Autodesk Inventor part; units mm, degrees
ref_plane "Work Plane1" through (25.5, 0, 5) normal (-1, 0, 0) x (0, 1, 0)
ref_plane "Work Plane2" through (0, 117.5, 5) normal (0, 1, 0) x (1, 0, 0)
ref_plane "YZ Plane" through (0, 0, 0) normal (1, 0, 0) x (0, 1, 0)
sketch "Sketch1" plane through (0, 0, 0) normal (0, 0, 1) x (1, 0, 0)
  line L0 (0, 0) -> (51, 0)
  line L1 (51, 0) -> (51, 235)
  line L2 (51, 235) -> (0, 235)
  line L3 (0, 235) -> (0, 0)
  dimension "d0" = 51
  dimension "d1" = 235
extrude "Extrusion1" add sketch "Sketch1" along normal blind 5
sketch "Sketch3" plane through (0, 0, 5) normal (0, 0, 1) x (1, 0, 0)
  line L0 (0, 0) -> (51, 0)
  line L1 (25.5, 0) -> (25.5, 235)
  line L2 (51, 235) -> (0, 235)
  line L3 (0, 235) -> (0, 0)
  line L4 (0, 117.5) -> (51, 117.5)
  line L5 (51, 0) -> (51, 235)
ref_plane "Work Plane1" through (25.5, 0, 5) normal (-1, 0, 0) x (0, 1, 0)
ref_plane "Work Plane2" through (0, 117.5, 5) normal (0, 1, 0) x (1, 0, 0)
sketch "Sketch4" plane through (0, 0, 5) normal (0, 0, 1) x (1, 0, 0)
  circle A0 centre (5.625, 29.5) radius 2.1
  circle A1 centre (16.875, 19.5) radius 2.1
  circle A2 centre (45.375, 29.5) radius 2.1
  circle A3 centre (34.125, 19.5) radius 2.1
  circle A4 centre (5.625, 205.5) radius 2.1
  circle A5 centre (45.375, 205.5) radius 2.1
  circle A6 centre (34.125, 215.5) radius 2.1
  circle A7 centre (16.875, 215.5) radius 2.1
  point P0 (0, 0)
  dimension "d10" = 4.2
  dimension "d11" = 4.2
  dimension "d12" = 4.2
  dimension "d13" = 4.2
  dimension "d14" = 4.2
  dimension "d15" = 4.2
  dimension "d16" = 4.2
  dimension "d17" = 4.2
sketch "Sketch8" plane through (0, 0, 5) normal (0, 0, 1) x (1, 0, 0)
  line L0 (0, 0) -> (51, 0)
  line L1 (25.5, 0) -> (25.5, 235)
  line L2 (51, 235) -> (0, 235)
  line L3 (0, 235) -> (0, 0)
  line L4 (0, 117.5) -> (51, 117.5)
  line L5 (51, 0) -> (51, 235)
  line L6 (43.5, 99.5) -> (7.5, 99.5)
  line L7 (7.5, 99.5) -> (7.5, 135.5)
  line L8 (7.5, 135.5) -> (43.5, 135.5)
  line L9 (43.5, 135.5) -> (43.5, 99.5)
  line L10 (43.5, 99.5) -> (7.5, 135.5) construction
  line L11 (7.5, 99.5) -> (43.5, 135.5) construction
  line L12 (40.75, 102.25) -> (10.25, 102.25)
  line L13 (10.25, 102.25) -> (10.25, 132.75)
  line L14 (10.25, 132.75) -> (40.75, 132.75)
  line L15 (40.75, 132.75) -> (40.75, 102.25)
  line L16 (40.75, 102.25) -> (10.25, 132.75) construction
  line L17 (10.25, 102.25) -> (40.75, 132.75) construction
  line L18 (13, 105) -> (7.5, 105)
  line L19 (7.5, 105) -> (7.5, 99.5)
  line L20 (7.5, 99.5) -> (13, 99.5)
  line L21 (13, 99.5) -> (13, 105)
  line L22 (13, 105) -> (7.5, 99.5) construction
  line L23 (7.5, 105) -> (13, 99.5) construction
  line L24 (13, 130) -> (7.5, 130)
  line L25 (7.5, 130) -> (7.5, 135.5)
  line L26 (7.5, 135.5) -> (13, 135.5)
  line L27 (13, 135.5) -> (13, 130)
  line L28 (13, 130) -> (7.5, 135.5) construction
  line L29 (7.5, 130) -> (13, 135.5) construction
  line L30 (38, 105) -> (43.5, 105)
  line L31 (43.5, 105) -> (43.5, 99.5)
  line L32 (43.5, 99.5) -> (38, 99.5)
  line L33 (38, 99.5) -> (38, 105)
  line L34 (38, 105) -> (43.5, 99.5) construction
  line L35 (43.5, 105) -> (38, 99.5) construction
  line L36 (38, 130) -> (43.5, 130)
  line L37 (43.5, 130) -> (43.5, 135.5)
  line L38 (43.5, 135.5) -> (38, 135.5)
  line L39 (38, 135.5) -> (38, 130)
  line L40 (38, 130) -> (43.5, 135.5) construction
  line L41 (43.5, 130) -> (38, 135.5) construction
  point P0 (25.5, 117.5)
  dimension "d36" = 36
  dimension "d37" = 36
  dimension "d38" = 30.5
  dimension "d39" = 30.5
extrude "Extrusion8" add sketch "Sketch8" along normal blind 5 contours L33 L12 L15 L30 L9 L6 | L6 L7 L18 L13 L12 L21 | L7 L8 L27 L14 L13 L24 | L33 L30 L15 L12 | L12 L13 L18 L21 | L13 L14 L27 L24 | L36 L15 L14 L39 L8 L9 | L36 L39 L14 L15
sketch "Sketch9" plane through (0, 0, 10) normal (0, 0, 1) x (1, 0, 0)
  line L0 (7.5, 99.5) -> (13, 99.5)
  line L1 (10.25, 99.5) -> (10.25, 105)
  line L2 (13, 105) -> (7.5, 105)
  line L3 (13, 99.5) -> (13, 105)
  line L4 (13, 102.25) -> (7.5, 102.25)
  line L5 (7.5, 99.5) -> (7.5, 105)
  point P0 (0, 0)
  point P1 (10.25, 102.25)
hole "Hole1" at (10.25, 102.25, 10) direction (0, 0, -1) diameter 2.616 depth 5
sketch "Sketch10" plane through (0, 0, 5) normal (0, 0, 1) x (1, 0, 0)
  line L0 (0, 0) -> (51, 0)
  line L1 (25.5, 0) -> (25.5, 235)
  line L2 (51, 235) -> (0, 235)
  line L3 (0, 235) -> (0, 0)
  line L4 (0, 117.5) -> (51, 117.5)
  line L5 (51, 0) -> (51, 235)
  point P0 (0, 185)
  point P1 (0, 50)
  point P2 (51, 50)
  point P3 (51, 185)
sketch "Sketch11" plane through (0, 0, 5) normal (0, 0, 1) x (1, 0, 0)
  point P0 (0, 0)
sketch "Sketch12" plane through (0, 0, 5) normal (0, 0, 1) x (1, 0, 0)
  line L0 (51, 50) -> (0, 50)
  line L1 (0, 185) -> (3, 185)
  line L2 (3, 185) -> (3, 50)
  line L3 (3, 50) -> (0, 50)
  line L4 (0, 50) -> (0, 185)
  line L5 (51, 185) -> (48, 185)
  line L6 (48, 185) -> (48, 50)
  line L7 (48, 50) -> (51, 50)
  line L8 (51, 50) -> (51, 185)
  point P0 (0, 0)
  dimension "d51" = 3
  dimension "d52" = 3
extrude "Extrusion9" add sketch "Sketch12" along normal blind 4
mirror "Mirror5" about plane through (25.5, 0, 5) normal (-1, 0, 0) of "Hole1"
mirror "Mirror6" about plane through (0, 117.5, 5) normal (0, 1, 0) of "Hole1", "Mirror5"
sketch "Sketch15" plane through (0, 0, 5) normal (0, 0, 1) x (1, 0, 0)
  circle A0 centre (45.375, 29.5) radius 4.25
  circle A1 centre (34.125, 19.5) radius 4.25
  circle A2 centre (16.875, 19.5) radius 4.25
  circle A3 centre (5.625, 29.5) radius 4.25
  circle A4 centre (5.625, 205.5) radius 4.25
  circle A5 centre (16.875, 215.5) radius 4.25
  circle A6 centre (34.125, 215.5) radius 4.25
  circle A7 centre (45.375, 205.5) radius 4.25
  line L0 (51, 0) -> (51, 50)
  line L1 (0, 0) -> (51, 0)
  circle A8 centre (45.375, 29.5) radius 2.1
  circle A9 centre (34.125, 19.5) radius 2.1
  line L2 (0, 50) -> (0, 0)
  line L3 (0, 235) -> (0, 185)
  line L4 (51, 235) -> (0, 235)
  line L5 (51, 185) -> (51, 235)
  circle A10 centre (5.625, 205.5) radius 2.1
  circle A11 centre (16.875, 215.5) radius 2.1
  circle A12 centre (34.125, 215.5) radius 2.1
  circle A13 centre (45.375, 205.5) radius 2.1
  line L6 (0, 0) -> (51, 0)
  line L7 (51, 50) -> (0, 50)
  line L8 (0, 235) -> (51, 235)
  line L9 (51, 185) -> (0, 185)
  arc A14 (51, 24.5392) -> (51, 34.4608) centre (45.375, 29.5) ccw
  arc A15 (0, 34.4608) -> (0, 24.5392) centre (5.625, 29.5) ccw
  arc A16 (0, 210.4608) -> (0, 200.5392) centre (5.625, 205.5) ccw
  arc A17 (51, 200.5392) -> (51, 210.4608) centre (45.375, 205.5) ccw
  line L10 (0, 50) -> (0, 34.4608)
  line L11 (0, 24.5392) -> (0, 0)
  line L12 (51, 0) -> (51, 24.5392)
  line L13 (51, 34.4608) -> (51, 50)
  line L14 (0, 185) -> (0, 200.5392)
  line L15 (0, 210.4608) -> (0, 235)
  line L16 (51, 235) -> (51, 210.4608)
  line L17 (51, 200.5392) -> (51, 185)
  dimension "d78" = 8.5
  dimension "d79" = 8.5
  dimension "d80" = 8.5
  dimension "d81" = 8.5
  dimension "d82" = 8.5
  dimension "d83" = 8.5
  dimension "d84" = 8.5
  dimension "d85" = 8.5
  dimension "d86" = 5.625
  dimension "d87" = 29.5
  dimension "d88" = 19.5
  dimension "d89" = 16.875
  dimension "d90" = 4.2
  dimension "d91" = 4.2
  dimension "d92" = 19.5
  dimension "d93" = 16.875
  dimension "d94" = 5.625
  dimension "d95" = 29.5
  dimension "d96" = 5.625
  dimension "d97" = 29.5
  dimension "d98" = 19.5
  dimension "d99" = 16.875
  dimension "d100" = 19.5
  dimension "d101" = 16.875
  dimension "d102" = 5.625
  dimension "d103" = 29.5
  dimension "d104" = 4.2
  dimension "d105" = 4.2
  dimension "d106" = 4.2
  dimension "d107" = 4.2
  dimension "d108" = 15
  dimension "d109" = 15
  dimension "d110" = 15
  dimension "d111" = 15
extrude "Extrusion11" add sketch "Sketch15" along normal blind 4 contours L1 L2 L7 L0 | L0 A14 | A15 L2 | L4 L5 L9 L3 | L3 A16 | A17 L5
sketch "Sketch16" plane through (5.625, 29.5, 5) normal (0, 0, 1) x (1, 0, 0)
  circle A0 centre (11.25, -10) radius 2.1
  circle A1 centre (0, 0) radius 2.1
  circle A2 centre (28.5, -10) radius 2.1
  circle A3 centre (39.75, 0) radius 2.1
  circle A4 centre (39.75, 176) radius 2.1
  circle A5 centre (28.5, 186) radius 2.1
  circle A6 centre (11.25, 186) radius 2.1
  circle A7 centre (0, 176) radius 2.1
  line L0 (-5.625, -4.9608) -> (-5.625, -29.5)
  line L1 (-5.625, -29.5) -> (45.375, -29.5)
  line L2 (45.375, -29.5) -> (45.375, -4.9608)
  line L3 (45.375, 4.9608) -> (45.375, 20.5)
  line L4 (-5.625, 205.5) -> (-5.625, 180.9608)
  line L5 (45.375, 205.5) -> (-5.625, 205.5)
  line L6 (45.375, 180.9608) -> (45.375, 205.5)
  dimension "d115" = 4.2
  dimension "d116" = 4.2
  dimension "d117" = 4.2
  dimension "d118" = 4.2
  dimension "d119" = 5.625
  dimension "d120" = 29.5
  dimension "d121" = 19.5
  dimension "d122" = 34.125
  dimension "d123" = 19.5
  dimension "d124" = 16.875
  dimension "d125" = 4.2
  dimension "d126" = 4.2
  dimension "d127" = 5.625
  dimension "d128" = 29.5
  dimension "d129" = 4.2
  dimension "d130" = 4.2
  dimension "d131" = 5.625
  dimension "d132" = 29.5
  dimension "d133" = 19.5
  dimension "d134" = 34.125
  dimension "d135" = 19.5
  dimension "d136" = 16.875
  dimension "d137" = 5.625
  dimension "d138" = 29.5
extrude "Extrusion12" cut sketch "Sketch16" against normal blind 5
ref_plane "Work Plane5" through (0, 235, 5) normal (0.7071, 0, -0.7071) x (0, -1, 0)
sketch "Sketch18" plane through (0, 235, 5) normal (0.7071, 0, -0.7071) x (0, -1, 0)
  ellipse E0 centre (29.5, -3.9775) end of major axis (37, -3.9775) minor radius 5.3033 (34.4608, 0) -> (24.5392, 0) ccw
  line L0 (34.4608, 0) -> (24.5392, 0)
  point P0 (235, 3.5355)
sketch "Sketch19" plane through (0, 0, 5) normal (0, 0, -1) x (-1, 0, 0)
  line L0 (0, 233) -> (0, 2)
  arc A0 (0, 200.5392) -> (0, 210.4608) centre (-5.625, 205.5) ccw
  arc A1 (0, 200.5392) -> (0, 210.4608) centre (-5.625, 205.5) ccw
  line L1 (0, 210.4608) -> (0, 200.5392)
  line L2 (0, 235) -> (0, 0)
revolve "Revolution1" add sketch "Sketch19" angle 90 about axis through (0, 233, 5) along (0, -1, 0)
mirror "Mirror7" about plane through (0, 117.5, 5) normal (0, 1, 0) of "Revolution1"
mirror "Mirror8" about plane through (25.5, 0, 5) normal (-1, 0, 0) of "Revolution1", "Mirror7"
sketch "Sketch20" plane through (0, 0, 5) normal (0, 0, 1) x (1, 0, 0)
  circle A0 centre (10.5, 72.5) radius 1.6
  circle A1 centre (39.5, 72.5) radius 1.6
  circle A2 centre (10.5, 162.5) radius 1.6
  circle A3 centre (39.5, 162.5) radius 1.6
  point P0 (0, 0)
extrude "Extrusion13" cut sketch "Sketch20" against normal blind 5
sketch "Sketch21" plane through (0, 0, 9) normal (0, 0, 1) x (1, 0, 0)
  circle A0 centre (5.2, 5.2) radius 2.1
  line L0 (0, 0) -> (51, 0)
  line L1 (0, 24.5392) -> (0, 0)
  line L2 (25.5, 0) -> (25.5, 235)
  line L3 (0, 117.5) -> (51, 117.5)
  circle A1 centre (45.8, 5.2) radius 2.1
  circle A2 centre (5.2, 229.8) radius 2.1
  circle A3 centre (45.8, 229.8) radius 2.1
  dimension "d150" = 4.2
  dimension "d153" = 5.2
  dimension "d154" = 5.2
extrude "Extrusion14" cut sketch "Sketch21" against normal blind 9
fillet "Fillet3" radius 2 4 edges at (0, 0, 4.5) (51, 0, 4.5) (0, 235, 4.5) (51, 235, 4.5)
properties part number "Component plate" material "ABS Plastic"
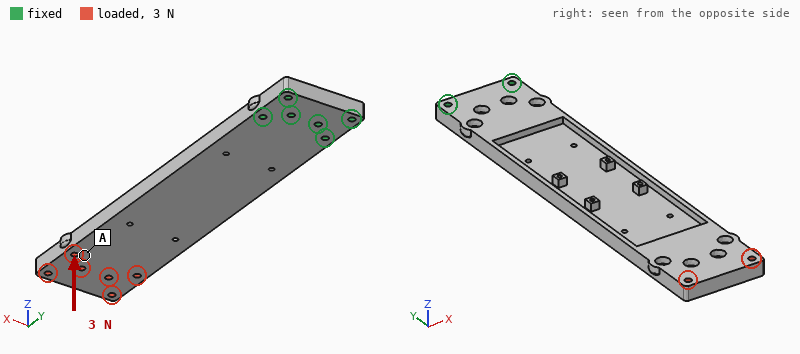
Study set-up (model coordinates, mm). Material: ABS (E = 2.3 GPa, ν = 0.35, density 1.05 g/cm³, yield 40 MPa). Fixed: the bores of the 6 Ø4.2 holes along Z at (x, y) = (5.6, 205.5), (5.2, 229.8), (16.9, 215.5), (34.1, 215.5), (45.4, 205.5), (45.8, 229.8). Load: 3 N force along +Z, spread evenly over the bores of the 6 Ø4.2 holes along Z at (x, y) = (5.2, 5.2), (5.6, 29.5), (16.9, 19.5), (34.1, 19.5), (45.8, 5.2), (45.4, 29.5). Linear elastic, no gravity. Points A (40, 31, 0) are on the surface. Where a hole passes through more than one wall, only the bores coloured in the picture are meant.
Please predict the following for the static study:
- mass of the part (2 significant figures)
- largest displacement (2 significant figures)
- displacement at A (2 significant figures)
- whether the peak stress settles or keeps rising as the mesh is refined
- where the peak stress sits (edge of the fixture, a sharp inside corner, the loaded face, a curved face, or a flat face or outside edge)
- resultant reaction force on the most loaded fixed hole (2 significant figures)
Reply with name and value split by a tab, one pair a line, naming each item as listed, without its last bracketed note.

mass of the part	85 g
largest displacement	2.9 mm
displacement at A	2.2 mm
whether the peak stress settles or keeps rising as the mesh is refined	keeps rising
where the peak stress sits	edge of the fixture
resultant reaction force on the most loaded fixed hole	17 N
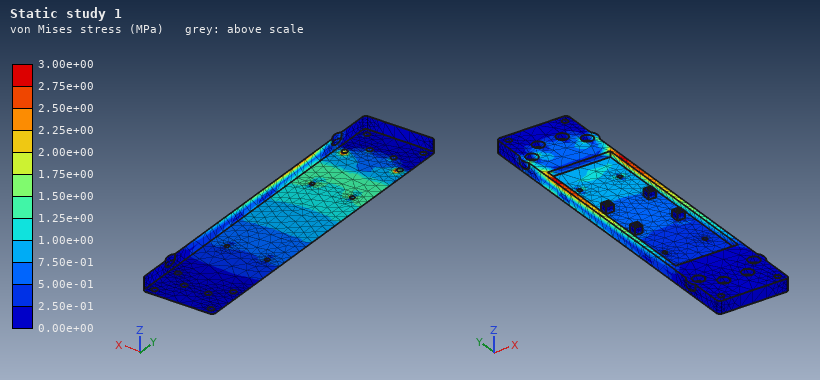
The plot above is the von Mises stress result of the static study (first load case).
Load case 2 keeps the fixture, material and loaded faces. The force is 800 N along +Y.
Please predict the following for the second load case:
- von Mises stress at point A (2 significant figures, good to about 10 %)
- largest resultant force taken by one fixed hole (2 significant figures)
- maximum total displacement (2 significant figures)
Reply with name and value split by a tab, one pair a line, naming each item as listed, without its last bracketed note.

von Mises stress at point A	2.8 MPa
largest resultant force taken by one fixed hole	230 N
maximum total displacement	2.9 mm
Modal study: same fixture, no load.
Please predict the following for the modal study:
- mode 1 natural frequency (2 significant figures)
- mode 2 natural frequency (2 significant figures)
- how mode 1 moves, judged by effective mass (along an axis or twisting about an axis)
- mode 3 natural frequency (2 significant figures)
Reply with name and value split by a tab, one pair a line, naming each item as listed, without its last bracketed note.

mode 1 natural frequency	35 Hz
mode 2 natural frequency	200 Hz
how mode 1 moves, judged by effective mass	along Z
mode 3 natural frequency	240 Hz
